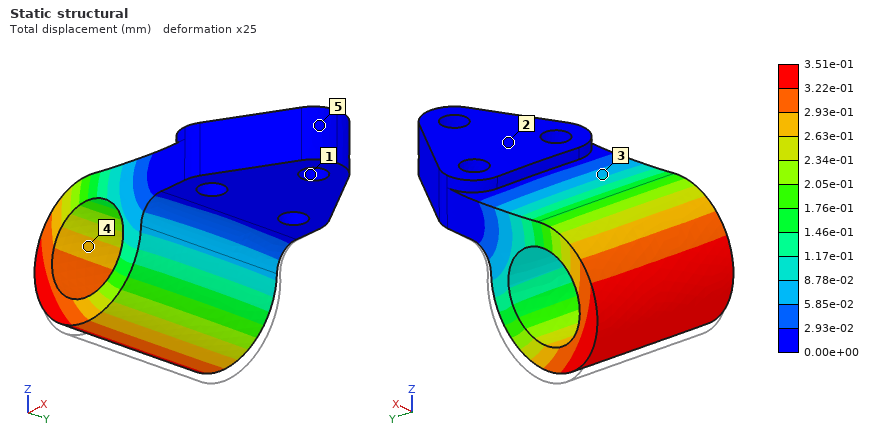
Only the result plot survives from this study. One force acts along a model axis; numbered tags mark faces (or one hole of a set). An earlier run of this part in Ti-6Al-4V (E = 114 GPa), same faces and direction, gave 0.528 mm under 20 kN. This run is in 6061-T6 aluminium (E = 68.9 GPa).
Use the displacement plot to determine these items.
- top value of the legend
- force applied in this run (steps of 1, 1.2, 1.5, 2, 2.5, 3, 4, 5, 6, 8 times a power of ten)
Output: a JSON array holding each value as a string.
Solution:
["3.51e-01 mm", "8 kN"]
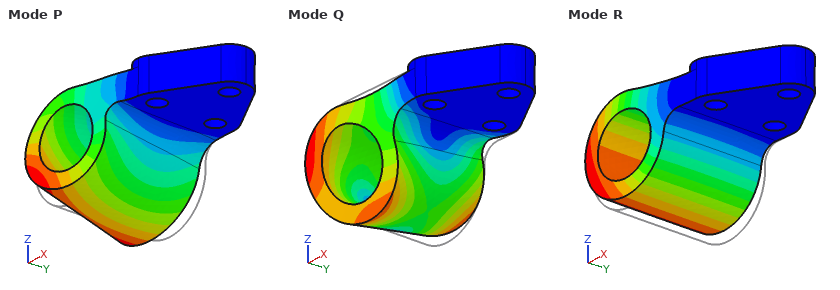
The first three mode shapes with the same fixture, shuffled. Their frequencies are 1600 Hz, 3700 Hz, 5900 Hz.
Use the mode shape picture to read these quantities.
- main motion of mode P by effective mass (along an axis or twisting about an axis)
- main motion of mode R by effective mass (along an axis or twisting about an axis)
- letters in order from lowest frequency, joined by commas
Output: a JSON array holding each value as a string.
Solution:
["along Y", "along Z", "R, P, Q"]
